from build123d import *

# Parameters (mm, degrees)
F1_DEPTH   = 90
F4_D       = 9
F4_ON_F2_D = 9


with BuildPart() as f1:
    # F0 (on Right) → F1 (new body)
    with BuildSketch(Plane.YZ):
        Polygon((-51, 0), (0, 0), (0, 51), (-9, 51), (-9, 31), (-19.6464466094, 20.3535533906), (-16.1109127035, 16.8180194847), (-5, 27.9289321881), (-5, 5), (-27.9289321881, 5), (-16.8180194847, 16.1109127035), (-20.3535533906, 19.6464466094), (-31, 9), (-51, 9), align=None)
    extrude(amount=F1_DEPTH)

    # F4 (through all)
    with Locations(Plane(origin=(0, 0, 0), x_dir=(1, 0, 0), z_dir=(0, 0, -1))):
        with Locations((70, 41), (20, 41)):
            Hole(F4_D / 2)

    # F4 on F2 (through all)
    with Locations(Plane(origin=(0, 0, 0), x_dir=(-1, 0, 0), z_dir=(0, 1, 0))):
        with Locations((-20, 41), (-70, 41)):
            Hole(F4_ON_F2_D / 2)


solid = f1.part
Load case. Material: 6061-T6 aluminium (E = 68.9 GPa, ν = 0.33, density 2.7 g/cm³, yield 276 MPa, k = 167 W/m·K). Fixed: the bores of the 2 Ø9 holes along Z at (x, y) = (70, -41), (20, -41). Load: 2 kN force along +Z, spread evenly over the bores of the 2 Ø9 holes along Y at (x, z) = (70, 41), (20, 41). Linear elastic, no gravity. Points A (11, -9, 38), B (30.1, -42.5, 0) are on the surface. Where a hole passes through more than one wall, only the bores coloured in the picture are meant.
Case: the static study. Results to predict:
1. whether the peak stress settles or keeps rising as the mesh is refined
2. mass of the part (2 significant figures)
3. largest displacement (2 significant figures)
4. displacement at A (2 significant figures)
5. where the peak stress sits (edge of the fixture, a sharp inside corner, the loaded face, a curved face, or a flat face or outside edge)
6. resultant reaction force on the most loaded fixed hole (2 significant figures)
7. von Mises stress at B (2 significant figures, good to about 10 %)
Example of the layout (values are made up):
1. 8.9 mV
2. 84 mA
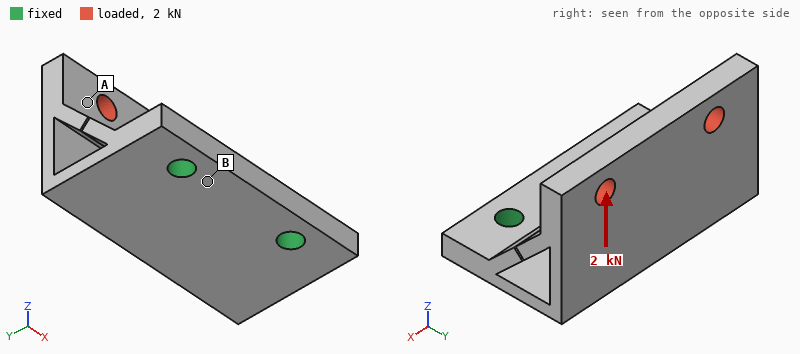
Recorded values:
1. keeps rising
2. 190 g
3. 0.55 mm
4. 0.40 mm
5. edge of the fixture
6. 1.0 kN
7. 25 MPa
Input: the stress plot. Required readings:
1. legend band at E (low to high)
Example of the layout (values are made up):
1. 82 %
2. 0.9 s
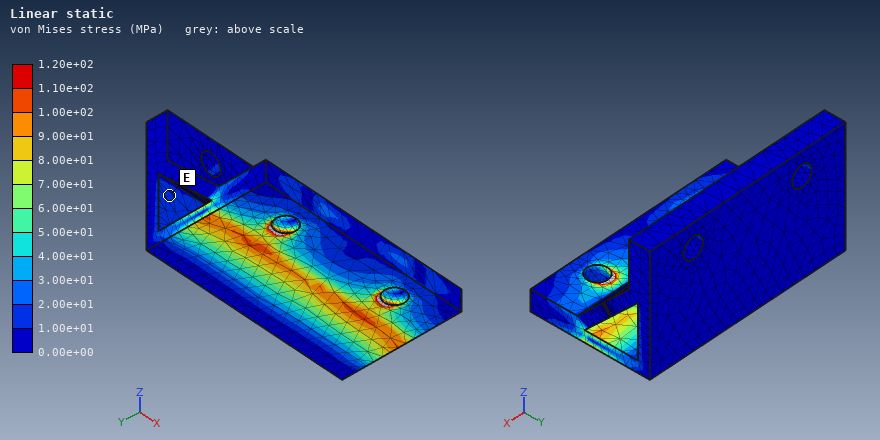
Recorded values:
1. 1.00e+01 to 2.00e+01 MPa
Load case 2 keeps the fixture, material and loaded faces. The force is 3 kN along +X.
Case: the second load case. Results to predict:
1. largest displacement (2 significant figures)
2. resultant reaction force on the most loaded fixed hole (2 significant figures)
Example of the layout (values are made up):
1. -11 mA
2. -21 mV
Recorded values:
1. 0.70 mm
2. 3.1 kN
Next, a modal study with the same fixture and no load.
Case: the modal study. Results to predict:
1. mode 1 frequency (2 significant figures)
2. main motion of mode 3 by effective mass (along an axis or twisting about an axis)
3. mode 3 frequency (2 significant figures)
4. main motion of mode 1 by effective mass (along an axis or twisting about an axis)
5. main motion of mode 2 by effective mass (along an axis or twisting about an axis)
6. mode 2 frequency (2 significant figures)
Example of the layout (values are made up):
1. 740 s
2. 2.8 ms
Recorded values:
1. 710 Hz
2. along Z
3. 1900 Hz
4. along Y
5. along X
6. 1300 Hz
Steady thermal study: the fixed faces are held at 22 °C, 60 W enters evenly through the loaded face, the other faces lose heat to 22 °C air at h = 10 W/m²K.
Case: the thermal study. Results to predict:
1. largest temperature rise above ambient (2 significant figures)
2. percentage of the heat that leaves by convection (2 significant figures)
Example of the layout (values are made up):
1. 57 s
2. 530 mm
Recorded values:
1. 53 K
2. 11 %
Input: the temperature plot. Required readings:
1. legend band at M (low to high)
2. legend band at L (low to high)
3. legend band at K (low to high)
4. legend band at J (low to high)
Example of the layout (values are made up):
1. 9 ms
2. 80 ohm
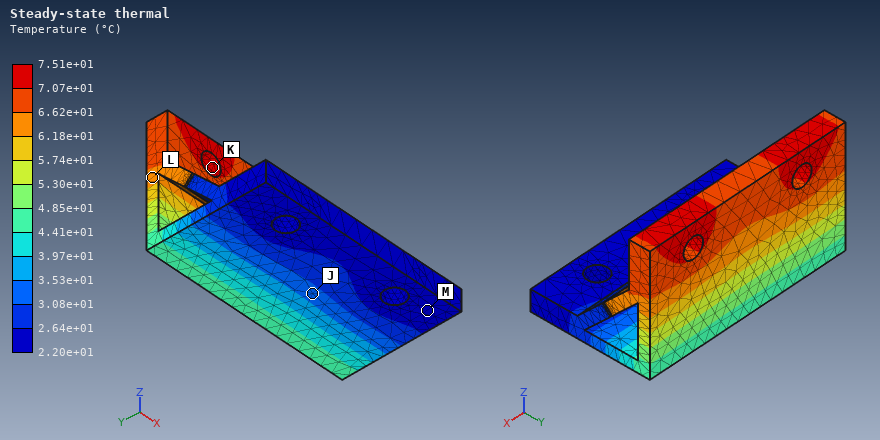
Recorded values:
1. 2.20e+01 to 2.64e+01 °C
2. 6.18e+01 to 6.62e+01 °C
3. 7.07e+01 to 7.51e+01 °C
4. 3.08e+01 to 3.53e+01 °C
